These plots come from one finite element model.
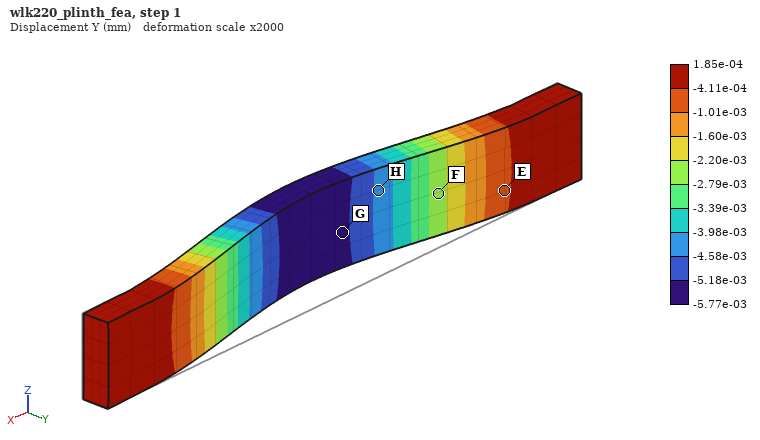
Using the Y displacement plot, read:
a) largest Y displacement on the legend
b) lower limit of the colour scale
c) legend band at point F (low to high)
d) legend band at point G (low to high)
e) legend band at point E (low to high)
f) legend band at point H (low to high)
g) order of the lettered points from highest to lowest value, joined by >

1.85e-04 mm
-5.77e-03 mm
-2.79e-03 to -2.20e-03 mm
-5.77e-03 to -5.18e-03 mm
-1.01e-03 to -4.11e-04 mm
-4.58e-03 to -3.98e-03 mm
E > F > H > G
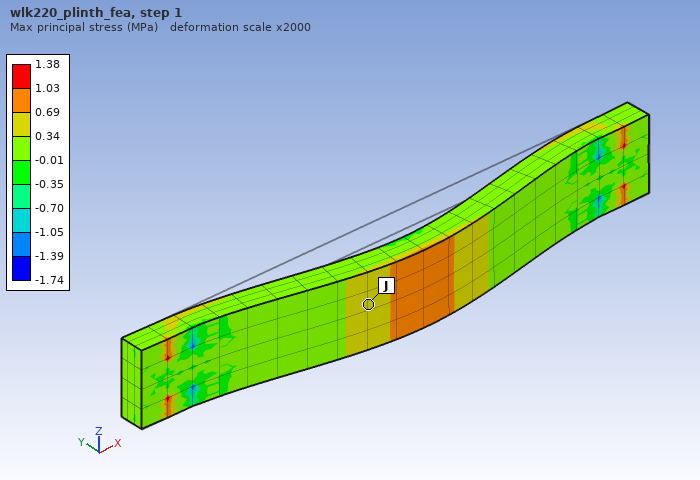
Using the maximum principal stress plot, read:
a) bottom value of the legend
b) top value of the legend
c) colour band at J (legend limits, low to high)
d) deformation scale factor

-1.74 MPa
1.38 MPa
0.34 to 0.69 MPa
2000
